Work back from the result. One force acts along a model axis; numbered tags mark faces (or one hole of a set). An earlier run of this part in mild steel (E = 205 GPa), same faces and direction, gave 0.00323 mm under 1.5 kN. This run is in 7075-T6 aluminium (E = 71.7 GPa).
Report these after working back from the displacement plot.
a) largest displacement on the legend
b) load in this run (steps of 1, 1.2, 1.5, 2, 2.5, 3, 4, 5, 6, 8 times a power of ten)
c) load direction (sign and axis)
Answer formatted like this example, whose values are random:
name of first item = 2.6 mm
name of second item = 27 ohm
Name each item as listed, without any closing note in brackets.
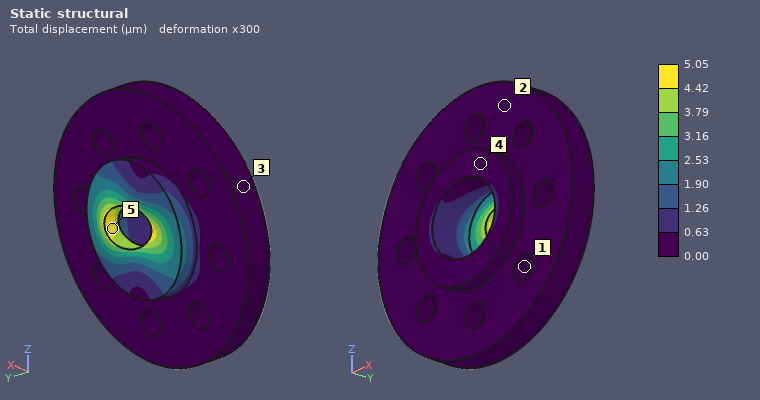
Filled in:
largest displacement on the legend = 5.05 µm
load in this run = 800 N
load direction = +X
